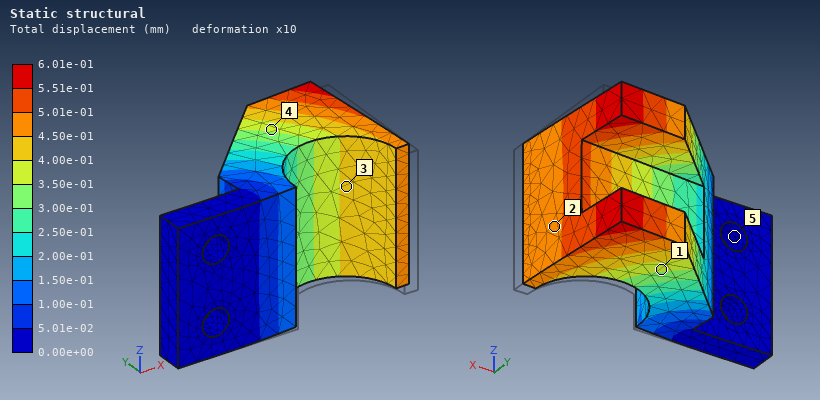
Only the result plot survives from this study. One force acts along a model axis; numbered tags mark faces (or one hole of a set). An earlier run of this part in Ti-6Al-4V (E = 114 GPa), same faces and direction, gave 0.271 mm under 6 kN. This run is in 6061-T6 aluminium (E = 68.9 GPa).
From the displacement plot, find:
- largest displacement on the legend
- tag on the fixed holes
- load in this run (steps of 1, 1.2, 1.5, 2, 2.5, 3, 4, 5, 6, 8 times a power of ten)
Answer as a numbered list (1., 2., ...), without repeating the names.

1. 6.01e-01 mm
2. 5
3. 8 kN
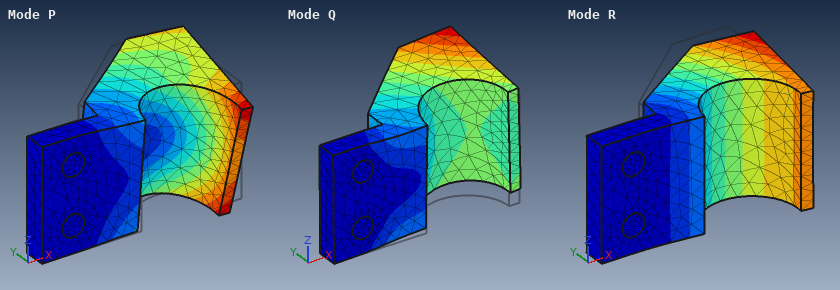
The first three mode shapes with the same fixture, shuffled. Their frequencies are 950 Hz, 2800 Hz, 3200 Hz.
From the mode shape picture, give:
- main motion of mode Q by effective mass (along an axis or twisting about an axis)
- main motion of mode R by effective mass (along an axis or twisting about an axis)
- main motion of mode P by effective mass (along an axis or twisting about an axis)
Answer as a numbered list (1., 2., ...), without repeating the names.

1. along Z
2. along Y
3. twisting about X
